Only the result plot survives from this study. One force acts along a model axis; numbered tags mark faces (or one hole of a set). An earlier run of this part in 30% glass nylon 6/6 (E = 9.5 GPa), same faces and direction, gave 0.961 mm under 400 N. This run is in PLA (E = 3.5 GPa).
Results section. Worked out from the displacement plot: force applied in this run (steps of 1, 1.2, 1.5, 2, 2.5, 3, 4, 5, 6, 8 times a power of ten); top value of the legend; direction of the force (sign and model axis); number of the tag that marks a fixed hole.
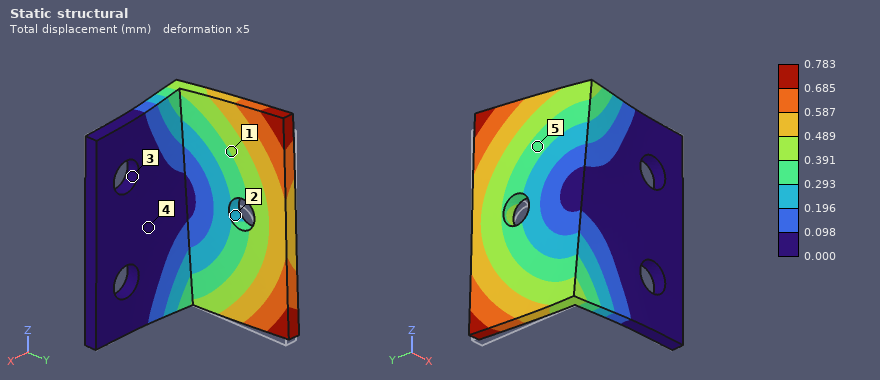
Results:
120 N
0.783 mm
+Z
3
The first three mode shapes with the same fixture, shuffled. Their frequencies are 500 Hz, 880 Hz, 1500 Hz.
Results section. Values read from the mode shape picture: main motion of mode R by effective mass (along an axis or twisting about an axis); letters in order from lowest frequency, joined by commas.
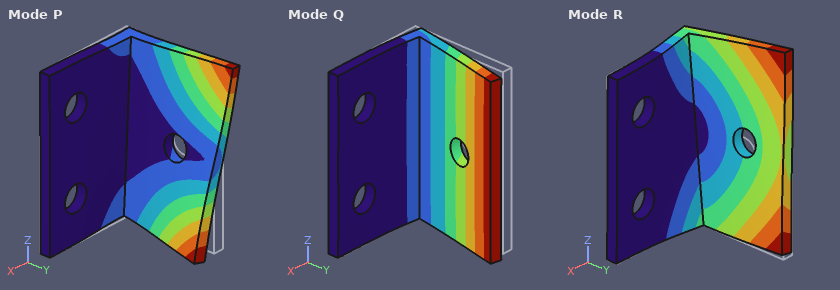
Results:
along Z
Q, R, P
